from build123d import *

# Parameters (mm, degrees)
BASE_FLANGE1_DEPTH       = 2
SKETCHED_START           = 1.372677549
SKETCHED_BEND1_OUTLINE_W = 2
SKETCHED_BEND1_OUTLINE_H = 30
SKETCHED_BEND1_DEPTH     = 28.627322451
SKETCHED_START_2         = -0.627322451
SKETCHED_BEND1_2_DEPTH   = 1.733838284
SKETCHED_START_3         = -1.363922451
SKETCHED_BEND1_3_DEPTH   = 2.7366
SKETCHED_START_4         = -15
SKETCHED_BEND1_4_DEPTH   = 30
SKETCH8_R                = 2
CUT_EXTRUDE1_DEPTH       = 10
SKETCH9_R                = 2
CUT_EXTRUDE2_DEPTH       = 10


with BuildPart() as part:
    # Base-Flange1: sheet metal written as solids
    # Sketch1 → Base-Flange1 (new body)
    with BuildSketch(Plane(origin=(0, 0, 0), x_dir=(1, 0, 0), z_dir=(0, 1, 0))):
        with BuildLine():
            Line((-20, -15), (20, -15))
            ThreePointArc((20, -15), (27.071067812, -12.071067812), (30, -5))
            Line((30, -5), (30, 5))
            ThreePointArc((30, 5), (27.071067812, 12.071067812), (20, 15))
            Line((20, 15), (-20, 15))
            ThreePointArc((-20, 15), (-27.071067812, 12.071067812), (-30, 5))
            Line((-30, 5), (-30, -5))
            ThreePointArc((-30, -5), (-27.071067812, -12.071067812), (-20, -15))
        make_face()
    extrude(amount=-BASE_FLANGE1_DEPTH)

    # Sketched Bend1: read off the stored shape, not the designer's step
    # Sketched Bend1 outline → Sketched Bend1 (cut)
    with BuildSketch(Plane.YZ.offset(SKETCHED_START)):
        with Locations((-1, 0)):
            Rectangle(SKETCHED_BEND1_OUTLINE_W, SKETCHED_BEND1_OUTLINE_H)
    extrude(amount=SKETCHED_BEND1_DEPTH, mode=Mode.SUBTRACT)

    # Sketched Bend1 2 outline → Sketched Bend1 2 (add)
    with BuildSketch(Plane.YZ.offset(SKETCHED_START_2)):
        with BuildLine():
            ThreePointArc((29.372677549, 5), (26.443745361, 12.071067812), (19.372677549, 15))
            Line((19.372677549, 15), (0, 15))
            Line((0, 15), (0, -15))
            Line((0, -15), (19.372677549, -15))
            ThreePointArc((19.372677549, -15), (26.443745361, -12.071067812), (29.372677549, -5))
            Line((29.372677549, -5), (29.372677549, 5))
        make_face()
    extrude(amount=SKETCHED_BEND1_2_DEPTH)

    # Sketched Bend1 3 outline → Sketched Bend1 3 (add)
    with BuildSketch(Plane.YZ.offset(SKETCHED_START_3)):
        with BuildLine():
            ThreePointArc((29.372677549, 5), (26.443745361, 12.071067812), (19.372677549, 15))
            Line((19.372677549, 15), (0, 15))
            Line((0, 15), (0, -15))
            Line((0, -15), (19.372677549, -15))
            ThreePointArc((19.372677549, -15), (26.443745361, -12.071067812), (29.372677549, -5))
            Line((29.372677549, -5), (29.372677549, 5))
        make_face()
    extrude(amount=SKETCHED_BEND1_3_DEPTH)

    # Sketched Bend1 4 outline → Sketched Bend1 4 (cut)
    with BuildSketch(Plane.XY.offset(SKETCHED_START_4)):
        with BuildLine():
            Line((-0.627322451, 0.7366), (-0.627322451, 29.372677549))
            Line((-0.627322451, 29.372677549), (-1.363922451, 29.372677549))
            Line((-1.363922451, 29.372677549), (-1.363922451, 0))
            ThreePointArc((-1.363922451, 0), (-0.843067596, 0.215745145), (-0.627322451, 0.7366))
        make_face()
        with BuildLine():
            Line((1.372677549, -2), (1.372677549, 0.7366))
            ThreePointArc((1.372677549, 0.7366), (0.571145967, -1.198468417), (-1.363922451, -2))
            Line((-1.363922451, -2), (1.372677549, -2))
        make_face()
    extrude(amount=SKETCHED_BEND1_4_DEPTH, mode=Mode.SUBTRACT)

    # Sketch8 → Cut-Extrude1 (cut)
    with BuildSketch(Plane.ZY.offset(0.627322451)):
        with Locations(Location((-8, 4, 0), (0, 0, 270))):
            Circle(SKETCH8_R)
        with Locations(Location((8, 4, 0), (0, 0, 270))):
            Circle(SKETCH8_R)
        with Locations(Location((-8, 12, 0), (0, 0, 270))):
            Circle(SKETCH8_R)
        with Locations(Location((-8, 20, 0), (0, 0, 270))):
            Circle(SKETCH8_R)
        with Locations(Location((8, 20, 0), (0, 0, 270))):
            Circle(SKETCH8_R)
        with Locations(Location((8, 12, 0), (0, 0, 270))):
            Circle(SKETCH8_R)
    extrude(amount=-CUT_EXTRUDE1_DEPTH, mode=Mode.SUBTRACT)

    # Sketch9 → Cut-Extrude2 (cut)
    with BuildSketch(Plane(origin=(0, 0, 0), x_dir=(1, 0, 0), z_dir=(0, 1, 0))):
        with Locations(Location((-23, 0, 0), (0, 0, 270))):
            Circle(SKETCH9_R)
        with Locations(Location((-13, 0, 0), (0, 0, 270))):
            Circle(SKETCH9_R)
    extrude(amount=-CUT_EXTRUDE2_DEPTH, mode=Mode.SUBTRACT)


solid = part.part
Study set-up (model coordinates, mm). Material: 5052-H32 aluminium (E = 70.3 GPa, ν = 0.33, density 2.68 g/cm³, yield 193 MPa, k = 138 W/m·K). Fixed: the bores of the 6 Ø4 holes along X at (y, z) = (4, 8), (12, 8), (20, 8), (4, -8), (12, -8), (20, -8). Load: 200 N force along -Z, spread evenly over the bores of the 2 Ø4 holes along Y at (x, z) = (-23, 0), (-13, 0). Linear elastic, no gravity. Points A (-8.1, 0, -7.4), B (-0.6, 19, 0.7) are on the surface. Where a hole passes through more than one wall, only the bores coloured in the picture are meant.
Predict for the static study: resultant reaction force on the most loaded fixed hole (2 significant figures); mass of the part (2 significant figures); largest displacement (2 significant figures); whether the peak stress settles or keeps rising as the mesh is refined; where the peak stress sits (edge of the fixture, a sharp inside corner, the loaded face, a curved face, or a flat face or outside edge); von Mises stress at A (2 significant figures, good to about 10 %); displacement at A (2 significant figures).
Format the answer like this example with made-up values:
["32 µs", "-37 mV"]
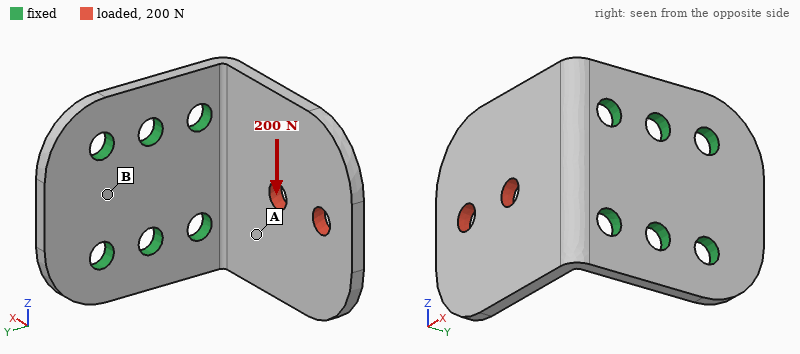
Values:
["240 N", "8.6 g", "34 µm", "keeps rising", "edge of the fixture", "15 MPa", "13 µm"]
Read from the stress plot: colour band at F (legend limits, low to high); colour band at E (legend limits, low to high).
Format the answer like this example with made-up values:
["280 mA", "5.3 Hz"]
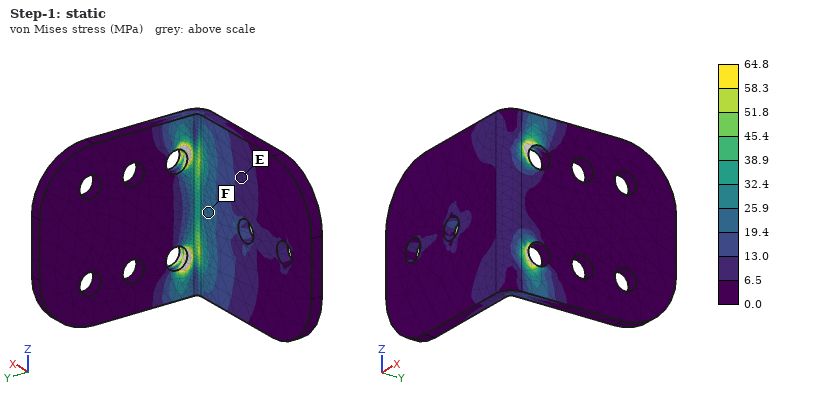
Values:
["19.4 to 25.9 MPa", "6.5 to 13.0 MPa"]
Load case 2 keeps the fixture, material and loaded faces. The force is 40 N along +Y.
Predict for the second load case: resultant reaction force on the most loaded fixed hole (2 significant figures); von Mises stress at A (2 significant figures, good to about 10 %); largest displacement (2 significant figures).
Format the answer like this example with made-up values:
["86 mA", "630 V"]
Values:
["19 N", "19 MPa", "0.17 mm"]
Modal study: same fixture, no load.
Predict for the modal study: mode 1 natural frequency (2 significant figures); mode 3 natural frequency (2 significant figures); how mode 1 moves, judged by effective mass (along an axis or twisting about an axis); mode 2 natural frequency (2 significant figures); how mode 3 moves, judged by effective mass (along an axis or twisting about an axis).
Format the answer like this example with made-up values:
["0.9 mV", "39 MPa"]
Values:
["1700 Hz", "8300 Hz", "along Y", "4500 Hz", "along Z"]
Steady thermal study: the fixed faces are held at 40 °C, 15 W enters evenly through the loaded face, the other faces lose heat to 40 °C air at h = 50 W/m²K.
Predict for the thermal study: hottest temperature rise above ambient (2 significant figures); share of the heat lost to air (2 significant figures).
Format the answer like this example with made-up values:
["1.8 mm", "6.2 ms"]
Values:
["42 K", "16 %"]
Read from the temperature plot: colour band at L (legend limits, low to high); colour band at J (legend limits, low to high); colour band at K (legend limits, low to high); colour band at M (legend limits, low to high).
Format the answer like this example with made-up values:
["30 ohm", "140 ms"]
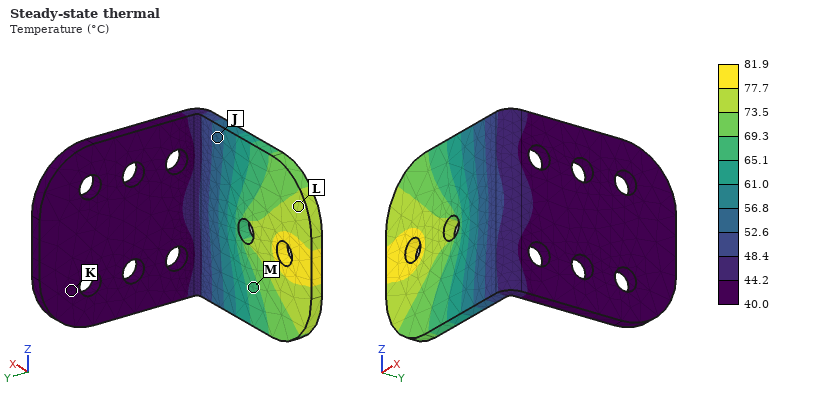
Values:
["73.5 to 77.7 °C", "52.6 to 56.8 °C", "40.0 to 44.2 °C", "65.1 to 69.3 °C"]
